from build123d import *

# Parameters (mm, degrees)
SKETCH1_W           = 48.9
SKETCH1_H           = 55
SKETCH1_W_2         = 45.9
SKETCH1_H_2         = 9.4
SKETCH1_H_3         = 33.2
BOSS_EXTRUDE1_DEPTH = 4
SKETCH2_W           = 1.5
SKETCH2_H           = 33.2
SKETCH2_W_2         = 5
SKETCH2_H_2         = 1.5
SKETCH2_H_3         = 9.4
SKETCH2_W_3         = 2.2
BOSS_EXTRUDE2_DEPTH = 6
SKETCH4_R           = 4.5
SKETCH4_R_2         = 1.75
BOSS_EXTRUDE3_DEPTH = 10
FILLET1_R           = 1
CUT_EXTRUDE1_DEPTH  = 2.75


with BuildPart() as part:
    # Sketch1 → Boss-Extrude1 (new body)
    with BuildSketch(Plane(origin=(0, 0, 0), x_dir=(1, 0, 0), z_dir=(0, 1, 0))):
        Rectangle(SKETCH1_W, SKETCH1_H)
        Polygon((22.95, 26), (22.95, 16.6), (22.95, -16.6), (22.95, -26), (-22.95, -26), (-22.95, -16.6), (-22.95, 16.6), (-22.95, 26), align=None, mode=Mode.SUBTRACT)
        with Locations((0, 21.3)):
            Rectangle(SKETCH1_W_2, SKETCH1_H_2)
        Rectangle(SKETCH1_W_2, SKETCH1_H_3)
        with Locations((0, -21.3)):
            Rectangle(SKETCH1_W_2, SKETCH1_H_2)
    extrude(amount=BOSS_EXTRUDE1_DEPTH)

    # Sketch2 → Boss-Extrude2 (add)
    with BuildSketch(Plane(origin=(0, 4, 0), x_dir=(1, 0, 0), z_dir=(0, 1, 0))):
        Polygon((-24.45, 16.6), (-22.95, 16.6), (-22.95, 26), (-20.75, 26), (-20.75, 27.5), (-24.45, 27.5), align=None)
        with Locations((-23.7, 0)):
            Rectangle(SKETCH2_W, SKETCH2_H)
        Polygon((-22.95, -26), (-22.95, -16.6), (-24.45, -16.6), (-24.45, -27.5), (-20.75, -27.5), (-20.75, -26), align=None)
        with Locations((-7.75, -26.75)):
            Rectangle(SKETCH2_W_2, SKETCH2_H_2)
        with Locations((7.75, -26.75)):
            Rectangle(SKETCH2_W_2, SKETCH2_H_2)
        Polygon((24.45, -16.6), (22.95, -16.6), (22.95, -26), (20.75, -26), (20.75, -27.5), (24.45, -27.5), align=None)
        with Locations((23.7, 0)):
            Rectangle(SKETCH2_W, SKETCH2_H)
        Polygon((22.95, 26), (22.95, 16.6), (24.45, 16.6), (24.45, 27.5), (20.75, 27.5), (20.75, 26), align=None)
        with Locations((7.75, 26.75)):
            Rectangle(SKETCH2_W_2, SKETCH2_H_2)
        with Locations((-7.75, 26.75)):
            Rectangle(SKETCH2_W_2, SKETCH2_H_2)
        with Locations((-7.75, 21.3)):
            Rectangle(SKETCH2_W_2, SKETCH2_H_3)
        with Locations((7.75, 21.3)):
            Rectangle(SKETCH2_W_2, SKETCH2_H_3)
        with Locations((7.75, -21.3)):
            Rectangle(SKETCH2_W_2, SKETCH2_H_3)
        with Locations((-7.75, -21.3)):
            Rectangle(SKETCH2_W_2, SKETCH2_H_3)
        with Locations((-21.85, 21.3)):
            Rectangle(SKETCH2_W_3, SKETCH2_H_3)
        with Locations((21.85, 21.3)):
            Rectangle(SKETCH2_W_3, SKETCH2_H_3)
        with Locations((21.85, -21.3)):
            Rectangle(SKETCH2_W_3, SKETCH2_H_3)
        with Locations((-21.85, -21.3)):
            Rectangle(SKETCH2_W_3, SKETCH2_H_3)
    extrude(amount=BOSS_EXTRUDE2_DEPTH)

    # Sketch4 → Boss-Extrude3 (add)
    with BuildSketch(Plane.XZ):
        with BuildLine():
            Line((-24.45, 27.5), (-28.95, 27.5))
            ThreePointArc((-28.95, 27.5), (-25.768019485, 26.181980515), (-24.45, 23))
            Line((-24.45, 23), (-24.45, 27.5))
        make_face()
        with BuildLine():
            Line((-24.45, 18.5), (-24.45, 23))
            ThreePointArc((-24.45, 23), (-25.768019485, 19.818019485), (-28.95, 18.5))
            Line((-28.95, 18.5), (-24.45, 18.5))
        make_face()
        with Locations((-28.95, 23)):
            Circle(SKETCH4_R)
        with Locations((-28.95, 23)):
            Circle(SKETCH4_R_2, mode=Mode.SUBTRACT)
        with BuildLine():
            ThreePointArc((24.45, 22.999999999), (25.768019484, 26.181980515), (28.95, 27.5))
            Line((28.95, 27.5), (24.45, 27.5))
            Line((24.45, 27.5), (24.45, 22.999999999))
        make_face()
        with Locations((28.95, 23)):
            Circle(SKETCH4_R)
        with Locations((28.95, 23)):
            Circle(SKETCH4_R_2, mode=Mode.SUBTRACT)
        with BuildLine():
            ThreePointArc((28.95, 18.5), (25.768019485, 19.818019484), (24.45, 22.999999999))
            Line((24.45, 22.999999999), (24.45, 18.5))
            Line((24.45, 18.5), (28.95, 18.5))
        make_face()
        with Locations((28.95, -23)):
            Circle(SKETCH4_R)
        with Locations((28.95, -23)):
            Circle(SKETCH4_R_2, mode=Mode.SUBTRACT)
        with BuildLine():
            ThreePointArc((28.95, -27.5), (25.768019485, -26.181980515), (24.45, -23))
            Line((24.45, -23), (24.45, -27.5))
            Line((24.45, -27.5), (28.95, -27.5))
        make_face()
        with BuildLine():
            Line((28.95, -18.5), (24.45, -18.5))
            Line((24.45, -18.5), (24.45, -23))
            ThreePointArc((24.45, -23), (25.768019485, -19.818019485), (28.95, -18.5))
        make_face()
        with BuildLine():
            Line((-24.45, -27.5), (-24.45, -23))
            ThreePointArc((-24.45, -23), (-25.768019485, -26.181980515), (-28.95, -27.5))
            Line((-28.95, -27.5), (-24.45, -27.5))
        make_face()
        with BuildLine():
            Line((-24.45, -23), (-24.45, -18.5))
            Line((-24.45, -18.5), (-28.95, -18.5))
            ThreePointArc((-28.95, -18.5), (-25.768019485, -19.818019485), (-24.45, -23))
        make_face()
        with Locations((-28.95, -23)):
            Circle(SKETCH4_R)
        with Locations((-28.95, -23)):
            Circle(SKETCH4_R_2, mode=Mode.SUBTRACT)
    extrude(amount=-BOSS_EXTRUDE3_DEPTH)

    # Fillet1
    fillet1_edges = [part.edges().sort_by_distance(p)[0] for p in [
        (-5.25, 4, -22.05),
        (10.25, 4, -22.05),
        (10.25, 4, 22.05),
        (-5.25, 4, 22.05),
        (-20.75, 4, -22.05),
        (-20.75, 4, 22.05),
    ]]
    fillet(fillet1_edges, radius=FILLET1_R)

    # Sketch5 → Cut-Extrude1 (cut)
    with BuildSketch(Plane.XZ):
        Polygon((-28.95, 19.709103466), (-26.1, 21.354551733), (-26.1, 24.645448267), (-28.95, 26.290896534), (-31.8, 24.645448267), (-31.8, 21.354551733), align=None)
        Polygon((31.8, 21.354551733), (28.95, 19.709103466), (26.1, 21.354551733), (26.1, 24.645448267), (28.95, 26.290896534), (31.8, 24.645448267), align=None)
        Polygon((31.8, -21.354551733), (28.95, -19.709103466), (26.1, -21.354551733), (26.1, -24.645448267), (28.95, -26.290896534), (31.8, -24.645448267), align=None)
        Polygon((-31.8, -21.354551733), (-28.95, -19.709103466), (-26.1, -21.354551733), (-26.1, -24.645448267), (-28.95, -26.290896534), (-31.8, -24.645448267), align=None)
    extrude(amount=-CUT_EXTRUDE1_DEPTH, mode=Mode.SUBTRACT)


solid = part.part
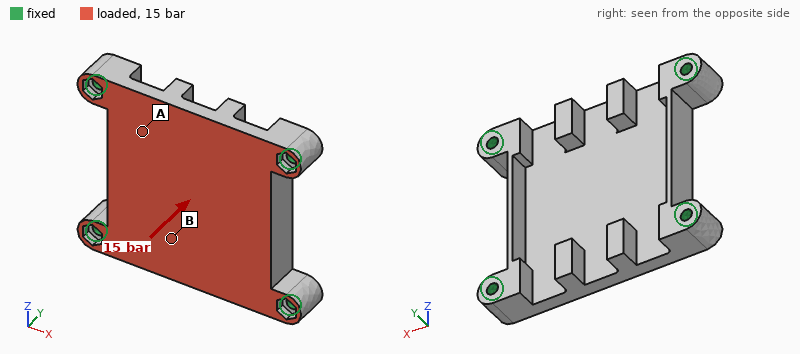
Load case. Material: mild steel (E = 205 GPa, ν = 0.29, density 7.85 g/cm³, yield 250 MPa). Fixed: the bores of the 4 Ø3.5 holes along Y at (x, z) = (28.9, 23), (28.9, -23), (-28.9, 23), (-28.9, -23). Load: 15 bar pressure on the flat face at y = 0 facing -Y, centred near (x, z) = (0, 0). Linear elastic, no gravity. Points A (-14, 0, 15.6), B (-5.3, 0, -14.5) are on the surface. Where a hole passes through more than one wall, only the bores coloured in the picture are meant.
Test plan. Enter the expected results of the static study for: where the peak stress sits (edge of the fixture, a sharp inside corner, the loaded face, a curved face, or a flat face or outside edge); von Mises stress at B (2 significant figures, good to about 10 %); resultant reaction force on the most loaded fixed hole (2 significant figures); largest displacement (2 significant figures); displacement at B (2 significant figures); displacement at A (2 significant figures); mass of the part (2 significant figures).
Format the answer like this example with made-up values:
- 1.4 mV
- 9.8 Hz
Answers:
- a curved face
- 61 MPa
- 1.5 kN
- 39 µm
- 31 µm
- 19 µm
- 130 g
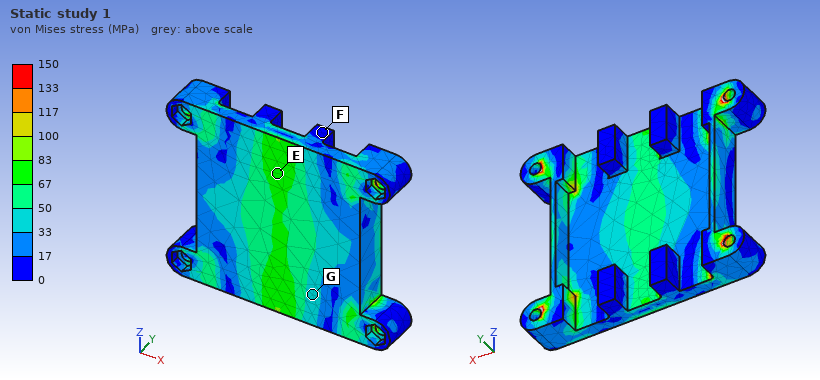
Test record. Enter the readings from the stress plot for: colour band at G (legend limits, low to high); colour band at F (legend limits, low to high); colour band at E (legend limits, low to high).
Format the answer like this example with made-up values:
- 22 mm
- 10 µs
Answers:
- 33 to 50 MPa
- 0 to 17 MPa
- 67 to 83 MPa
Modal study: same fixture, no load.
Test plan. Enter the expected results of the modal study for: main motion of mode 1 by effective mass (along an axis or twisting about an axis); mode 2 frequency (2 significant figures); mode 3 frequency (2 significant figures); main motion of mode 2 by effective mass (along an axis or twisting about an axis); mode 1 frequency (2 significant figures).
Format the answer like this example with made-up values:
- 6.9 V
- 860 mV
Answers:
- along Y
- 8400 Hz
- 11 kHz
- twisting about X
- 6300 Hz
